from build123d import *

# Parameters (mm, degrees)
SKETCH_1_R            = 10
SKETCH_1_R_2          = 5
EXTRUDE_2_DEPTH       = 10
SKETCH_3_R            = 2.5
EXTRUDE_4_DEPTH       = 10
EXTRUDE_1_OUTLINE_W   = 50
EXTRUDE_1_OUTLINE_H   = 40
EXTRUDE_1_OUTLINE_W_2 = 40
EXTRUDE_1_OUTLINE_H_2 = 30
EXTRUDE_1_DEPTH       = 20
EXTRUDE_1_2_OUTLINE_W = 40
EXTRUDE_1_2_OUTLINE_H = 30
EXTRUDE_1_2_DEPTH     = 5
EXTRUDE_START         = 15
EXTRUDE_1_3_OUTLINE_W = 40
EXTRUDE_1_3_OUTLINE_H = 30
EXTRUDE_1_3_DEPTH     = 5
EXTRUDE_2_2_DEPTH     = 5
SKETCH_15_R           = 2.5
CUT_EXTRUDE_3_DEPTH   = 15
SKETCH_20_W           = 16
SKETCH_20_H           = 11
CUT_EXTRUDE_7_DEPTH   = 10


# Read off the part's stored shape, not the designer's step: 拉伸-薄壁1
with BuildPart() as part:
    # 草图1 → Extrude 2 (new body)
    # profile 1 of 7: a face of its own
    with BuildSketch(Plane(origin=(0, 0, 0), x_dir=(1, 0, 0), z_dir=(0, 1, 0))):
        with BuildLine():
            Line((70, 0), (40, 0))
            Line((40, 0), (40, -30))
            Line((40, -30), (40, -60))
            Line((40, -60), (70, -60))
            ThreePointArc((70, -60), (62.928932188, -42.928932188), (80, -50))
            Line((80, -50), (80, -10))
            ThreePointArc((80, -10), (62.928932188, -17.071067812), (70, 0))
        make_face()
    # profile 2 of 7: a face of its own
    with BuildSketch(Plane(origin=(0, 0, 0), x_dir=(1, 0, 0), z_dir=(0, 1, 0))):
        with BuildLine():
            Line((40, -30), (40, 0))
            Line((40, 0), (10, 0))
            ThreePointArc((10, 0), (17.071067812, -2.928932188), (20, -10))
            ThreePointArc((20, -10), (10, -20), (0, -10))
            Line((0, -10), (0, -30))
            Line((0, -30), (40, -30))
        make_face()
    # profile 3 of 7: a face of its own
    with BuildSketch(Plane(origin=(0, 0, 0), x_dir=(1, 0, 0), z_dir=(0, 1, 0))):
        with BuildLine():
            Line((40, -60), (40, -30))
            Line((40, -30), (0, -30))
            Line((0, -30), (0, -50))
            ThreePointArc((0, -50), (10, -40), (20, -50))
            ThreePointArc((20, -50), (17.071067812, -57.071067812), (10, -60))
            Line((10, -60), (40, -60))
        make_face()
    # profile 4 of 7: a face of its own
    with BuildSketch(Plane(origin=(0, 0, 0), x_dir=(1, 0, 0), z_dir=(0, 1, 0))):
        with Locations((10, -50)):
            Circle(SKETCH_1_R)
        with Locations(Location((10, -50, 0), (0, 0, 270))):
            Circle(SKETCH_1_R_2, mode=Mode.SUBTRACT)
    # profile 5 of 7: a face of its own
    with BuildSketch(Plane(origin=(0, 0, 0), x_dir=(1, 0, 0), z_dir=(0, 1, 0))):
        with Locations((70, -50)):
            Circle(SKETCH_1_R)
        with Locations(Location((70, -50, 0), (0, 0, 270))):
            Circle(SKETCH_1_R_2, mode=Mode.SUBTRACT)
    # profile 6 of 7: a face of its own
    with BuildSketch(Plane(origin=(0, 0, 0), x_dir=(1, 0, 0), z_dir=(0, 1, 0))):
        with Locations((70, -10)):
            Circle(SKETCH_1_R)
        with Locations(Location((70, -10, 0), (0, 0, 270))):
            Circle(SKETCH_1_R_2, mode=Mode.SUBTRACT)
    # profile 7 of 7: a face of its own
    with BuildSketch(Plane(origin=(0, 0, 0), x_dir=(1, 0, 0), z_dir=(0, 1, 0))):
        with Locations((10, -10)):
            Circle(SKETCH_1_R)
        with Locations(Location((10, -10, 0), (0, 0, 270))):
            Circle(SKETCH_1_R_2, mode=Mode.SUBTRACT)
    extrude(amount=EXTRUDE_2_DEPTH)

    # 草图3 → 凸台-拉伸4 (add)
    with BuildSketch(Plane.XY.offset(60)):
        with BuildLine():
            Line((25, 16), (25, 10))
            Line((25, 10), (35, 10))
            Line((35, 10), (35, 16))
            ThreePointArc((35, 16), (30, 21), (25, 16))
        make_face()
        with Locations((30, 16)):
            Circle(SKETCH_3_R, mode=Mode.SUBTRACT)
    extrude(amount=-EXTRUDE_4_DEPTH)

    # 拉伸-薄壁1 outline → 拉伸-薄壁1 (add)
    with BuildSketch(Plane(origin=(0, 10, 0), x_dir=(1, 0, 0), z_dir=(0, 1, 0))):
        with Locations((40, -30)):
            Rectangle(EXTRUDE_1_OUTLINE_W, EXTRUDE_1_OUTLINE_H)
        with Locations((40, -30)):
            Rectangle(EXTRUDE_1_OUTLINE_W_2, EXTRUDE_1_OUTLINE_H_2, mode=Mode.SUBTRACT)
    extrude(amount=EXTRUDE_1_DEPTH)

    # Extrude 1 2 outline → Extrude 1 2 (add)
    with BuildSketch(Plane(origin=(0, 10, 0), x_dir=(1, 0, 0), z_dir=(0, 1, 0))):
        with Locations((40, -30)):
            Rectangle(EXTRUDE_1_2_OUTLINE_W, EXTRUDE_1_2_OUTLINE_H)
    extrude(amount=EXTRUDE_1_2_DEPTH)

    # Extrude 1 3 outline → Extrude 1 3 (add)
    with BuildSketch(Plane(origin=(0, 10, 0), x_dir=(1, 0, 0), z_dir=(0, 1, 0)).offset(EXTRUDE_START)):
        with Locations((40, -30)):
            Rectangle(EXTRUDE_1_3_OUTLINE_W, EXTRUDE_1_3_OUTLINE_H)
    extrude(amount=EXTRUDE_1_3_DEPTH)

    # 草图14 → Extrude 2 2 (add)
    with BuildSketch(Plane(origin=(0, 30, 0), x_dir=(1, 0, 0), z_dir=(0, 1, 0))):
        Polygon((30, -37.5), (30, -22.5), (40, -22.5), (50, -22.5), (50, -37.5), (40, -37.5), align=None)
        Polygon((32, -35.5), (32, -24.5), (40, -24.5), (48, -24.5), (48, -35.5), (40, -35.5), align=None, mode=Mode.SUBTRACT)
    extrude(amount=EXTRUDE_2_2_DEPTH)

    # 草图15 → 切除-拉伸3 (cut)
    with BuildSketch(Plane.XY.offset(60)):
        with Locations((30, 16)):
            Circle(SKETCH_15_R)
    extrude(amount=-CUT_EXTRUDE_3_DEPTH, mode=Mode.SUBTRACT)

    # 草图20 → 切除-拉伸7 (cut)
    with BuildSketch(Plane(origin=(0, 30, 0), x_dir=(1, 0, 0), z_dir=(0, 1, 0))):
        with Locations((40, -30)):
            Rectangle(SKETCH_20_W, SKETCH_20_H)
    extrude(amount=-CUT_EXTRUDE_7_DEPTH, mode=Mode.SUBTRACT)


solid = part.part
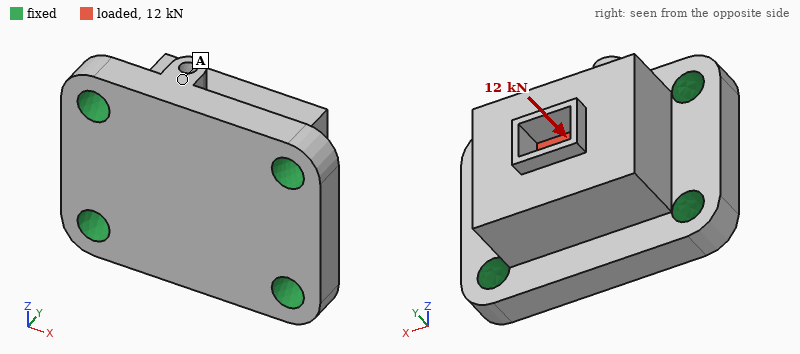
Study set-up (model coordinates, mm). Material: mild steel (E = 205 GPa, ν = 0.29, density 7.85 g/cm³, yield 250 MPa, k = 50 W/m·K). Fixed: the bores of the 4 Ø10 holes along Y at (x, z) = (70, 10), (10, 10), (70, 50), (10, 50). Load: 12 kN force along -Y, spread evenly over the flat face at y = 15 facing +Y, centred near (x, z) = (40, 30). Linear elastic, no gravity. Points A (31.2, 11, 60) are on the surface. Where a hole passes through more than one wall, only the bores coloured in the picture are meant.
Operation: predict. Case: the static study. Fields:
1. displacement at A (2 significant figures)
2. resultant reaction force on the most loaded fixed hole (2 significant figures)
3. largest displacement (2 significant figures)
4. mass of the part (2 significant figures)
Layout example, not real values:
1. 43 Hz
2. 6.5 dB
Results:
1. 2.5 µm
2. 3.3 kN
3. 5.9 µm
4. 570 g
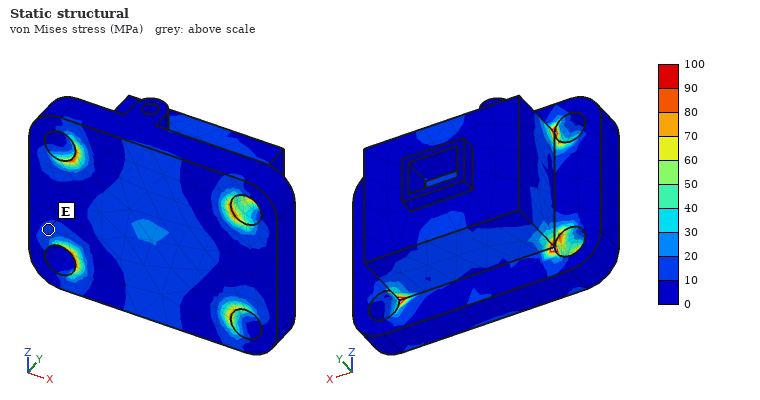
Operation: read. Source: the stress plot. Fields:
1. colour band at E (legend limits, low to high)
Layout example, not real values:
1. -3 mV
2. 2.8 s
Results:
1. 10 to 20 MPa
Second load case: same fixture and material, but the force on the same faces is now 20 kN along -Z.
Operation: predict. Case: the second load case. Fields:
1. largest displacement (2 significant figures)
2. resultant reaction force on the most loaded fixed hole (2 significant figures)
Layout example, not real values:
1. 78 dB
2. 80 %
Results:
1. 5.9 µm
2. 6.3 kN
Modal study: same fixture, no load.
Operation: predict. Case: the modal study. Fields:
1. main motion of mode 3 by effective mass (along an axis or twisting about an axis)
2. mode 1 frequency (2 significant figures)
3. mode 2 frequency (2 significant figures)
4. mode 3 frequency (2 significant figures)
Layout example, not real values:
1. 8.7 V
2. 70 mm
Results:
1. along X
2. 14 kHz
3. 15 kHz
4. 18 kHz
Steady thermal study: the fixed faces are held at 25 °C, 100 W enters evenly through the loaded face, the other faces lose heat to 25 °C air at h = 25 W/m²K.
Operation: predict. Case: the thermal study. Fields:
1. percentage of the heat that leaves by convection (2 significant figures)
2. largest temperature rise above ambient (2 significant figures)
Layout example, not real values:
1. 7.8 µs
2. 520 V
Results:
1. 7.1 %
2. 40 K
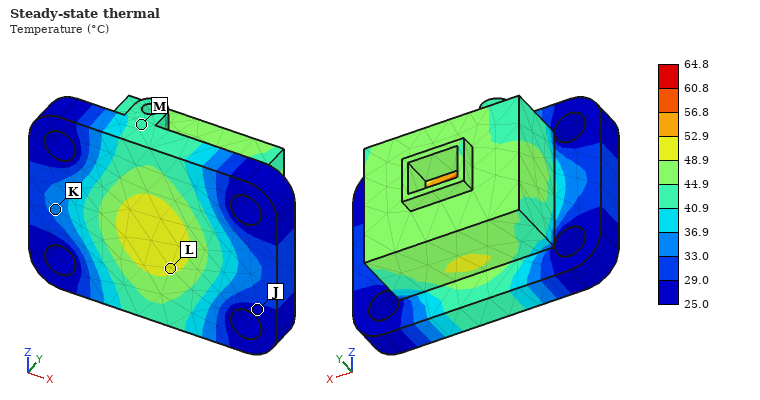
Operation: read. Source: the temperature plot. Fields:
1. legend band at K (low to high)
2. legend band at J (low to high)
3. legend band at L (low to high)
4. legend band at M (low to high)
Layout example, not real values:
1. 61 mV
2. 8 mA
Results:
1. 33.0 to 36.9 °C
2. 25.0 to 29.0 °C
3. 48.9 to 52.9 °C
4. 40.9 to 44.9 °C
